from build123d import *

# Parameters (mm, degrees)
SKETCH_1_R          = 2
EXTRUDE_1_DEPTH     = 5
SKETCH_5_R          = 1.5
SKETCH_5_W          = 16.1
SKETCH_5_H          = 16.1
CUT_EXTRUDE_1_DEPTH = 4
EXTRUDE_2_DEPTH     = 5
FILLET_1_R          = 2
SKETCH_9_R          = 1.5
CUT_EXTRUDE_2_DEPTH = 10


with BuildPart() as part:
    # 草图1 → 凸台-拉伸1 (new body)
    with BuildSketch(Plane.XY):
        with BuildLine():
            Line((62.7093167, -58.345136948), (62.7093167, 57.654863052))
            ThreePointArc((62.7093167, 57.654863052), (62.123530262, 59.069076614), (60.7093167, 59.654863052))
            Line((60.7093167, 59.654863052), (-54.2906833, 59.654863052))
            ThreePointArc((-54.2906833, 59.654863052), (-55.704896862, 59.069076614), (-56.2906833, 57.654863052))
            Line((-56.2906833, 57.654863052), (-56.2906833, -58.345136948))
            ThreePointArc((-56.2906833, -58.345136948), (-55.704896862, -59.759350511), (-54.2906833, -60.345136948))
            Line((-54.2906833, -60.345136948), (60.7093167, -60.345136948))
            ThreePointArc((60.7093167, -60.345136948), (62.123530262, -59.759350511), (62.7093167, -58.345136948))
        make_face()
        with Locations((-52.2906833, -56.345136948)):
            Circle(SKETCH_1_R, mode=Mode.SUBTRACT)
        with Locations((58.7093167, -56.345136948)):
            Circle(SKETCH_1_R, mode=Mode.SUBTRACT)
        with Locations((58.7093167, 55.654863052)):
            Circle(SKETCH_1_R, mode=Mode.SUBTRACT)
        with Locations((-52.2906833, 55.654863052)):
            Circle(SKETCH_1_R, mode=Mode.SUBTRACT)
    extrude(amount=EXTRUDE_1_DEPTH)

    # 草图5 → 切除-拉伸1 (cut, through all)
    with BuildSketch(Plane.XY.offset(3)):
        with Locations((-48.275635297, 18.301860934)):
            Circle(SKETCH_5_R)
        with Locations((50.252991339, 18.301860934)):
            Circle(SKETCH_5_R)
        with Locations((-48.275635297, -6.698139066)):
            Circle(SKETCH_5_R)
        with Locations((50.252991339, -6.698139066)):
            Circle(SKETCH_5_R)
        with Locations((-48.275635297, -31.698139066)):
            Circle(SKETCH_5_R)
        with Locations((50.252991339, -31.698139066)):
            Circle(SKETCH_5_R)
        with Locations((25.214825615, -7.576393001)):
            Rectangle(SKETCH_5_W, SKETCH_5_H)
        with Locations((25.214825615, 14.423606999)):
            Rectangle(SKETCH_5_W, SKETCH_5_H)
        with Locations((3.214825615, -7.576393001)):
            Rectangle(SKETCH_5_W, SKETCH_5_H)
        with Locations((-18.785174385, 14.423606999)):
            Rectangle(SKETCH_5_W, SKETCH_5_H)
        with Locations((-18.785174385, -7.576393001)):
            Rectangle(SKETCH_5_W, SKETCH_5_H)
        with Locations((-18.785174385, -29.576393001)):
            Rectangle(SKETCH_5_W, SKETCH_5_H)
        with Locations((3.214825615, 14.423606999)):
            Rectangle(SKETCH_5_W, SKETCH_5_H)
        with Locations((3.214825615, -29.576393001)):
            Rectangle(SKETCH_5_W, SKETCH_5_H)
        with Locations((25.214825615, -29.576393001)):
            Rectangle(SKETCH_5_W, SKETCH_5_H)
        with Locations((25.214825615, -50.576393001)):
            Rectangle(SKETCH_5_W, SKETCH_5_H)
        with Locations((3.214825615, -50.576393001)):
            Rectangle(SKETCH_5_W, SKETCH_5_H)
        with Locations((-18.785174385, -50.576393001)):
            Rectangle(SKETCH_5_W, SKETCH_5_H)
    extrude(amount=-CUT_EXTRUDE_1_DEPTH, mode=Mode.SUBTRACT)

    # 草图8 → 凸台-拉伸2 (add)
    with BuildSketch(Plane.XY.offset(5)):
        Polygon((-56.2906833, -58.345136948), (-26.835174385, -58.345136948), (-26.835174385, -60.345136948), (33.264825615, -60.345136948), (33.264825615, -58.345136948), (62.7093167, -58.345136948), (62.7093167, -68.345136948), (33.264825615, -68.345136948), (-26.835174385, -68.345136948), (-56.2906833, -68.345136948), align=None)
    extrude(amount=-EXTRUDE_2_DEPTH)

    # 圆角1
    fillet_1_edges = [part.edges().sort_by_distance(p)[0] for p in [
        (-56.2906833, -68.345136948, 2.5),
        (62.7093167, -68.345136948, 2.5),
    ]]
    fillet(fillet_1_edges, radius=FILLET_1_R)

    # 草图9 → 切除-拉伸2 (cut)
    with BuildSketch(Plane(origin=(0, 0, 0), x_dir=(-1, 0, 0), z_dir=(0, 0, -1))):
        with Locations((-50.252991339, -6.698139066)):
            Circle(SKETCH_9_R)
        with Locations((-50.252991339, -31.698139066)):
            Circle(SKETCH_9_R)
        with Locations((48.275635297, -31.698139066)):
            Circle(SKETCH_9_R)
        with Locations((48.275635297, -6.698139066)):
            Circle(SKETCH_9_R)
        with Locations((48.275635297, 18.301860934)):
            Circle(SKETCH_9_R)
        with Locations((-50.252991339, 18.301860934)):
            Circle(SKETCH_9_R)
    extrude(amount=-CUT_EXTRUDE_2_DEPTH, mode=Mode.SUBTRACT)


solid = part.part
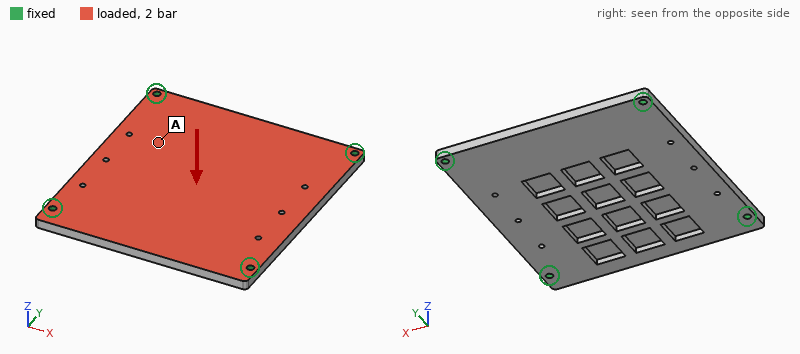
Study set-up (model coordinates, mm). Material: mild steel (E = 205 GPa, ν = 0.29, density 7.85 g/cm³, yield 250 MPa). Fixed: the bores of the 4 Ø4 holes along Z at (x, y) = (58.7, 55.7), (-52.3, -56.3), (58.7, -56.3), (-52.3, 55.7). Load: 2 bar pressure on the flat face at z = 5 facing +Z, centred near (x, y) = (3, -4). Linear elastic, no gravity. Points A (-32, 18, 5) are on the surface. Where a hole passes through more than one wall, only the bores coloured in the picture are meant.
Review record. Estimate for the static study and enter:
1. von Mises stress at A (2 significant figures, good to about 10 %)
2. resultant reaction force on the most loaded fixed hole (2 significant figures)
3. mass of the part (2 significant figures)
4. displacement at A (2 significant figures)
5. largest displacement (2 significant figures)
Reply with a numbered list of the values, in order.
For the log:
1. 30 MPa
2. 1.2 kN
3. 520 g
4. 0.11 mm
5. 0.17 mm
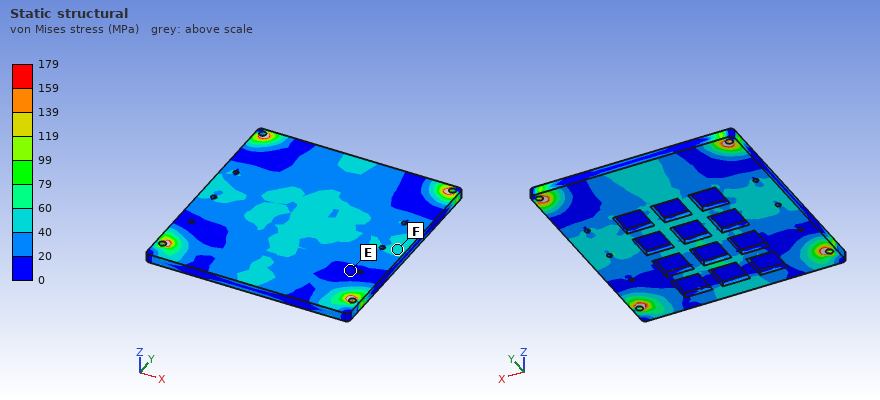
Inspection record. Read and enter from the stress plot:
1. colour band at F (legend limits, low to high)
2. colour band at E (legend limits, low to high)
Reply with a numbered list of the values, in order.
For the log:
1. 40 to 60 MPa
2. 0 to 20 MPa
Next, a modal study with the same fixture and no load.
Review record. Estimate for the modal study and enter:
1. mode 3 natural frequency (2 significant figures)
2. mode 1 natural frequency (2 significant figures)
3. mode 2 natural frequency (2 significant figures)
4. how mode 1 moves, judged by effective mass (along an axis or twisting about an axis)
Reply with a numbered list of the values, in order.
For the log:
1. 2200 Hz
2. 1200 Hz
3. 2100 Hz
4. along Z
